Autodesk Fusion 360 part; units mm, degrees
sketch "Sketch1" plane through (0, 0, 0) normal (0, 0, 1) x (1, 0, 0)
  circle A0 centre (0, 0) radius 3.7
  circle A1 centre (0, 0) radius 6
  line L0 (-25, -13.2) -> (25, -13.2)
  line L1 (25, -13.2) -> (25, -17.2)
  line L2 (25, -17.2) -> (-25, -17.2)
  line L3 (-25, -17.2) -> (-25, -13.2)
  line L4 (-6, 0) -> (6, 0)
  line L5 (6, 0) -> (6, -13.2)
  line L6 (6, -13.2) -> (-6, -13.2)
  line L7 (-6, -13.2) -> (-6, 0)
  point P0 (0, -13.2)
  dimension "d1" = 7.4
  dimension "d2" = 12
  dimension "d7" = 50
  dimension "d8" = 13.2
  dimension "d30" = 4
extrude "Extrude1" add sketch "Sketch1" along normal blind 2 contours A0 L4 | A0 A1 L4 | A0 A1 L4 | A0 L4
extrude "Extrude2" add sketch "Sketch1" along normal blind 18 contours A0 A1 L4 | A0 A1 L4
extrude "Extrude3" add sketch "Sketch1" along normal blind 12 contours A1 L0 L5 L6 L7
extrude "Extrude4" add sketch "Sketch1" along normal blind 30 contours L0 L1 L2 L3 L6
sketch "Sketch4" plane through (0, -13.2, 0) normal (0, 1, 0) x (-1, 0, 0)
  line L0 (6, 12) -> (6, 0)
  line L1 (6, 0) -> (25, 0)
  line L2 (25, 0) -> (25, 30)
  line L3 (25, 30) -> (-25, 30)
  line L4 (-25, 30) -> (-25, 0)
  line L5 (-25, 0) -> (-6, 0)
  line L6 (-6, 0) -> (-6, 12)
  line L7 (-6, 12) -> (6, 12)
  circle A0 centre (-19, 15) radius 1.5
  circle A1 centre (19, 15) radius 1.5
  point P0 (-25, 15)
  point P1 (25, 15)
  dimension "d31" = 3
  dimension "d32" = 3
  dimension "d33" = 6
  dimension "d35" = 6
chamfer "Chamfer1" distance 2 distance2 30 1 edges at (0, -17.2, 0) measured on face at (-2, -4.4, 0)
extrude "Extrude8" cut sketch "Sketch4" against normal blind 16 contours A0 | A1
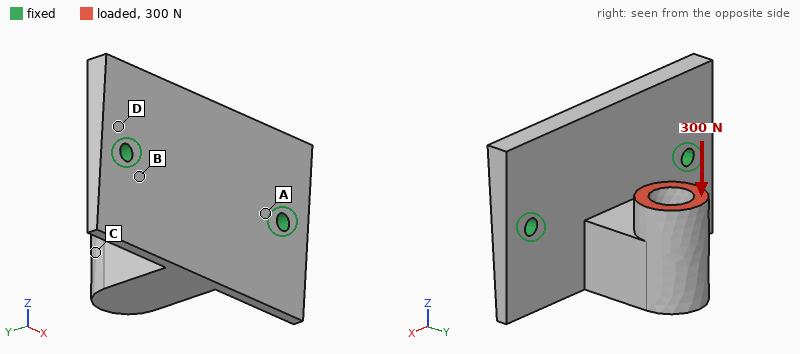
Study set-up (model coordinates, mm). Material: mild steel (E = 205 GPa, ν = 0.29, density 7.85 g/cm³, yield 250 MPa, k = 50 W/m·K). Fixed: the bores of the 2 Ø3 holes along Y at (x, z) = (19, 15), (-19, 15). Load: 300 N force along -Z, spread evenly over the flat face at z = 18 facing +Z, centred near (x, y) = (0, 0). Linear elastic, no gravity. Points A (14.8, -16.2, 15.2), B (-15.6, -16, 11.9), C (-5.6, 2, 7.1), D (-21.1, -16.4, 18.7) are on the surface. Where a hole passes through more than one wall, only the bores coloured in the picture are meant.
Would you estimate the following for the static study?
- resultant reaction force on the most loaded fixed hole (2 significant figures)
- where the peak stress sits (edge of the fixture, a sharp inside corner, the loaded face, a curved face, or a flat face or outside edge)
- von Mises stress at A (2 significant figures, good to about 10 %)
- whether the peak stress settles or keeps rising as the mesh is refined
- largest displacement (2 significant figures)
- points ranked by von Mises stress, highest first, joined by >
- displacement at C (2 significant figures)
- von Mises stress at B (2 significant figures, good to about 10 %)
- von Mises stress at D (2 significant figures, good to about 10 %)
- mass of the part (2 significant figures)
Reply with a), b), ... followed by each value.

a) 150 N
b) edge of the fixture
c) 44 MPa
d) keeps rising
e) 71 µm
f) B > A > D > C
g) 52 µm
h) 63 MPa
i) 31 MPa
j) 55 g
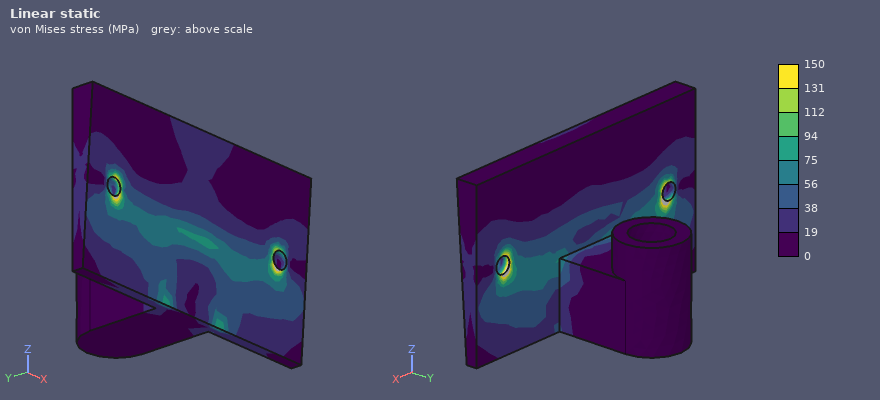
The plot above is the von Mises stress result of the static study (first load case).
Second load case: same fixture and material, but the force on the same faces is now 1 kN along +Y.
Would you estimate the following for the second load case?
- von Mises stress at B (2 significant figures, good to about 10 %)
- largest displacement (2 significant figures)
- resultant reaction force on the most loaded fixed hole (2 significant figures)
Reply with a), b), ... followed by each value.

a) 75 MPa
b) 89 µm
c) 500 N
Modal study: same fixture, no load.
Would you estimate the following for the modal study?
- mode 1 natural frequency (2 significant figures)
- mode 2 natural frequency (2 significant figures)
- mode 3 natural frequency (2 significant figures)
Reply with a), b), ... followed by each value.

a) 2900 Hz
b) 6200 Hz
c) 6300 Hz
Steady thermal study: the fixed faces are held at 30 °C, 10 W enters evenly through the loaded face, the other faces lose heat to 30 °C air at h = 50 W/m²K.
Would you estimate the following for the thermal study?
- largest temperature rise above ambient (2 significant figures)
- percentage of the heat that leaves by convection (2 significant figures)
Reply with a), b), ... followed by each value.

a) 61 K
b) 41 %
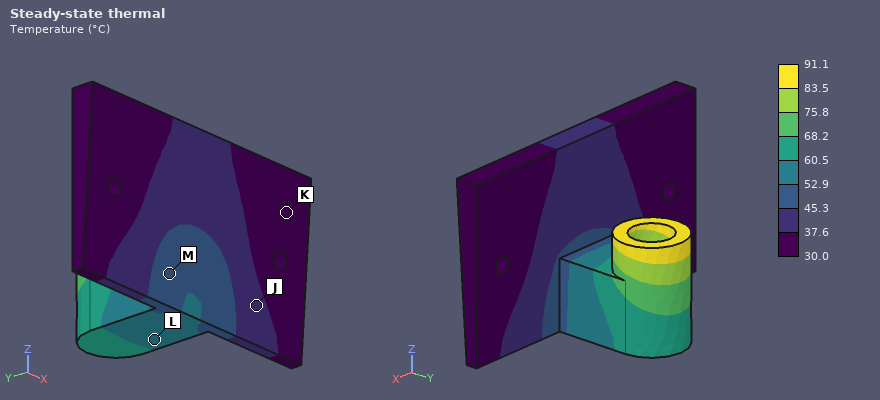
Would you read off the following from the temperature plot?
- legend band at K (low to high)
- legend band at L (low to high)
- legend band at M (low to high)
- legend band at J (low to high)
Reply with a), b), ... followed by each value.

a) 30.0 to 37.6 °C
b) 52.9 to 60.5 °C
c) 45.3 to 52.9 °C
d) 37.6 to 45.3 °C
